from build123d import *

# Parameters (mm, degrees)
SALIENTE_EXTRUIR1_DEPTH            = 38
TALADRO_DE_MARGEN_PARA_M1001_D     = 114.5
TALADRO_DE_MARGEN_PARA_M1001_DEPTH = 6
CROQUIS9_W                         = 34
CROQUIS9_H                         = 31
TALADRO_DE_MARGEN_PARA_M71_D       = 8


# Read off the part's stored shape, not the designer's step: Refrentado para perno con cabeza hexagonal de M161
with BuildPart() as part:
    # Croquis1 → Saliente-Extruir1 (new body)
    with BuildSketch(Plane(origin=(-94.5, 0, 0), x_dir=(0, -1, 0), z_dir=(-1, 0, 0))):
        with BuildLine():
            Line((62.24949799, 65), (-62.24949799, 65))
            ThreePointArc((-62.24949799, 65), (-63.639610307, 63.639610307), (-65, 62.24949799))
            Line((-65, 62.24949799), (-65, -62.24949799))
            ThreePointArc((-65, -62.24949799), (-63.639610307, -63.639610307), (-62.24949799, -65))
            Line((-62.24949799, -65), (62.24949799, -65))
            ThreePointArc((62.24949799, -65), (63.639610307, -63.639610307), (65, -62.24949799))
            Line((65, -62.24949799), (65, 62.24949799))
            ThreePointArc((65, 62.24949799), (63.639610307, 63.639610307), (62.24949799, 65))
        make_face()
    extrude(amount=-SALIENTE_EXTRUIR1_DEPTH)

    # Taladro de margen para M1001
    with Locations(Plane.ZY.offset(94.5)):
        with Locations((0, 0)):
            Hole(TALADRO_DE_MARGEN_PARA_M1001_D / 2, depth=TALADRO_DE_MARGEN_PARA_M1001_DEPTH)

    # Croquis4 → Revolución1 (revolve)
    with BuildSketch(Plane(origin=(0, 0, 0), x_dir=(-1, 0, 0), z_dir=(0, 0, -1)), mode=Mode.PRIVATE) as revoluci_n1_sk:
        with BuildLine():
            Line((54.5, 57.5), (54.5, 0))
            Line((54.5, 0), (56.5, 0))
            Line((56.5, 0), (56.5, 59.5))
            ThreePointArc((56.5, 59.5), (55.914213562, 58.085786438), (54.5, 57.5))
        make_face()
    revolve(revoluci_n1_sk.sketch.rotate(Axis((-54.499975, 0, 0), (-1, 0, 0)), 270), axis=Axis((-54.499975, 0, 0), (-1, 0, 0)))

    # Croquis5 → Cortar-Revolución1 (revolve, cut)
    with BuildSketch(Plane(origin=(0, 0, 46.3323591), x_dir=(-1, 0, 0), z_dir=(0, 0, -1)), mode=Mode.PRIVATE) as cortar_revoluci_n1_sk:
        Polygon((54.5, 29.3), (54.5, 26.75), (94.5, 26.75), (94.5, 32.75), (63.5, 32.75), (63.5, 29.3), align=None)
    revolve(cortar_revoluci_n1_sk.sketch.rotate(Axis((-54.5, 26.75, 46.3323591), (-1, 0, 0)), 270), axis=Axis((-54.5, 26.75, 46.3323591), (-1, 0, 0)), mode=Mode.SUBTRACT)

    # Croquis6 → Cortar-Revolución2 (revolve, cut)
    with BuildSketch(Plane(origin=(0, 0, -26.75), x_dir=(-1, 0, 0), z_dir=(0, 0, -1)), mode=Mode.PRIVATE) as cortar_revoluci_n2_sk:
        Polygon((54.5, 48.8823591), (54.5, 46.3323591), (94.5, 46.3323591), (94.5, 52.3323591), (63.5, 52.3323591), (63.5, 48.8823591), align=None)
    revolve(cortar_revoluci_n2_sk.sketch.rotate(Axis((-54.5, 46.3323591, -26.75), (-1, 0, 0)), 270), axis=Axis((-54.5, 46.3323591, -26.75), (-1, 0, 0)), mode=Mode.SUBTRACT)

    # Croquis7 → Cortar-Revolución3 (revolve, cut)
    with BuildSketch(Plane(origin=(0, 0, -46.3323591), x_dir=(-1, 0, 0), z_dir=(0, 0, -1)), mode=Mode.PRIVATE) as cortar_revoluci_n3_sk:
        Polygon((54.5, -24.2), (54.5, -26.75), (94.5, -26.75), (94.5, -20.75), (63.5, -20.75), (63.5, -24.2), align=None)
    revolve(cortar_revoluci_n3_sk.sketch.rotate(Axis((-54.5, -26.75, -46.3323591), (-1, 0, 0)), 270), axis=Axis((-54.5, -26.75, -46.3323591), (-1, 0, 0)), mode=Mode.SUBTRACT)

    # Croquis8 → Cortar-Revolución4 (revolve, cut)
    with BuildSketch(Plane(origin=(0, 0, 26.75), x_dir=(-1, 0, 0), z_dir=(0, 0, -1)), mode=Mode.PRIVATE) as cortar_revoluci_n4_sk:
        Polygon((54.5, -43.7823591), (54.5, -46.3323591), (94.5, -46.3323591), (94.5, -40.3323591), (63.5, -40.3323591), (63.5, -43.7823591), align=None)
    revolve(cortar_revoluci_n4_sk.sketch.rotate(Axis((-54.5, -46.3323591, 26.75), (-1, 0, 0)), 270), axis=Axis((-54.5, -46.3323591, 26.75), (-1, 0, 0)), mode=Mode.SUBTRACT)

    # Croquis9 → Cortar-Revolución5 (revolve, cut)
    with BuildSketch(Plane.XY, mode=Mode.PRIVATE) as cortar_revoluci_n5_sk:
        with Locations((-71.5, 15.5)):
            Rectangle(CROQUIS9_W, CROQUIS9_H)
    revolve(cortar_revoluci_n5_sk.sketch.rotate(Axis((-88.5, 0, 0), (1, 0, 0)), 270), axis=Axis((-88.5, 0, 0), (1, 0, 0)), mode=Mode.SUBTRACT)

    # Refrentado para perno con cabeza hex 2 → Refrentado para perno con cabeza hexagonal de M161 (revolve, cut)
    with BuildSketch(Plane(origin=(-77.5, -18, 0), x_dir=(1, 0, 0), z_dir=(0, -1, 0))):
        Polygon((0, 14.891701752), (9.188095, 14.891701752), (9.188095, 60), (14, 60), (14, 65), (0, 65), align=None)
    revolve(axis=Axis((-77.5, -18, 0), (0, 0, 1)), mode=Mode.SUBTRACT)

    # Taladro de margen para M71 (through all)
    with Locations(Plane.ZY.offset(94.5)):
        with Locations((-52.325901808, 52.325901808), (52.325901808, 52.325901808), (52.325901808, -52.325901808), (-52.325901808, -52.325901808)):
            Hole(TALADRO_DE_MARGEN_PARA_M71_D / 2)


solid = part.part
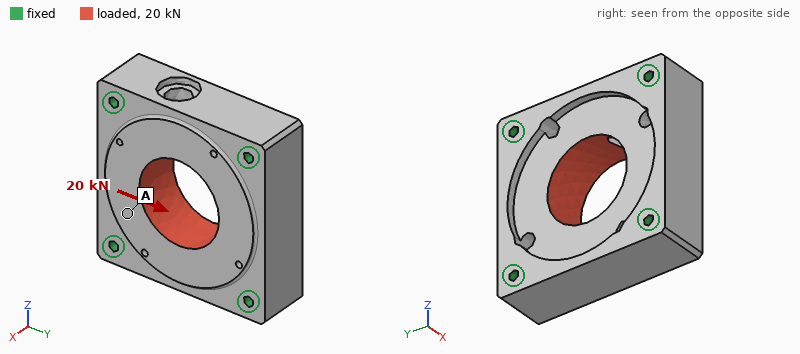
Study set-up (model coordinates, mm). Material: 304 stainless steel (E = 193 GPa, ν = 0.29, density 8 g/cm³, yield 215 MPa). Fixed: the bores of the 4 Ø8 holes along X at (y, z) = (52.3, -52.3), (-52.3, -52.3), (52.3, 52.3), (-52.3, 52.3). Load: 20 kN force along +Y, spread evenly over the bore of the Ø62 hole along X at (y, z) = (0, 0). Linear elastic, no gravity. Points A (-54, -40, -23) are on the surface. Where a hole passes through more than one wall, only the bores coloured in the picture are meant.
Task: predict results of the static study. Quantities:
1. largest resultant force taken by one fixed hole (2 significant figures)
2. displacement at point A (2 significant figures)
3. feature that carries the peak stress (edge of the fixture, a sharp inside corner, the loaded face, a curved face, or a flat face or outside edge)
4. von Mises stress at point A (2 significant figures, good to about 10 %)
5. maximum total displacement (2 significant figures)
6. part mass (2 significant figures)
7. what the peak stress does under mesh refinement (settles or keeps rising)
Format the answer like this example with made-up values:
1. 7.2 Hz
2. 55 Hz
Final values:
1. 5.9 kN
2. 1.6 µm
3. edge of the fixture
4. 4.2 MPa
5. 2.7 µm
6. 3.7 kg
7. keeps rising
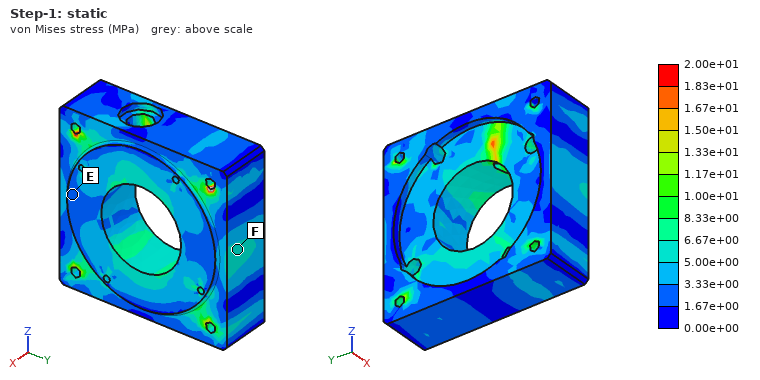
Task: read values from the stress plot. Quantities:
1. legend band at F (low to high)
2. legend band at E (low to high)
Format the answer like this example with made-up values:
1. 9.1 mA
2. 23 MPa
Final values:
1. 5.00e+00 to 6.67e+00 MPa
2. 1.67e+00 to 3.33e+00 MPa
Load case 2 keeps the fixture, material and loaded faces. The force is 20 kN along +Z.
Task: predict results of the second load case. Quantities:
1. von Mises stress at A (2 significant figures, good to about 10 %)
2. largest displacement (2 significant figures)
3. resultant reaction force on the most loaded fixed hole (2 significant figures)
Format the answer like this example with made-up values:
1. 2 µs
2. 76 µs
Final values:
1. 3.6 MPa
2. 2.5 µm
3. 5.8 kN
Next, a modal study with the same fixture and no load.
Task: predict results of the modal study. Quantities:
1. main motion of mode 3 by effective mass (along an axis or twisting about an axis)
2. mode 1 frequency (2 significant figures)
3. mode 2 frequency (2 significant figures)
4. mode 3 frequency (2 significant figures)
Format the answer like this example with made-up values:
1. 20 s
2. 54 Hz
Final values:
1. twisting about Y
2. 8100 Hz
3. 8300 Hz
4. 10 kHz
